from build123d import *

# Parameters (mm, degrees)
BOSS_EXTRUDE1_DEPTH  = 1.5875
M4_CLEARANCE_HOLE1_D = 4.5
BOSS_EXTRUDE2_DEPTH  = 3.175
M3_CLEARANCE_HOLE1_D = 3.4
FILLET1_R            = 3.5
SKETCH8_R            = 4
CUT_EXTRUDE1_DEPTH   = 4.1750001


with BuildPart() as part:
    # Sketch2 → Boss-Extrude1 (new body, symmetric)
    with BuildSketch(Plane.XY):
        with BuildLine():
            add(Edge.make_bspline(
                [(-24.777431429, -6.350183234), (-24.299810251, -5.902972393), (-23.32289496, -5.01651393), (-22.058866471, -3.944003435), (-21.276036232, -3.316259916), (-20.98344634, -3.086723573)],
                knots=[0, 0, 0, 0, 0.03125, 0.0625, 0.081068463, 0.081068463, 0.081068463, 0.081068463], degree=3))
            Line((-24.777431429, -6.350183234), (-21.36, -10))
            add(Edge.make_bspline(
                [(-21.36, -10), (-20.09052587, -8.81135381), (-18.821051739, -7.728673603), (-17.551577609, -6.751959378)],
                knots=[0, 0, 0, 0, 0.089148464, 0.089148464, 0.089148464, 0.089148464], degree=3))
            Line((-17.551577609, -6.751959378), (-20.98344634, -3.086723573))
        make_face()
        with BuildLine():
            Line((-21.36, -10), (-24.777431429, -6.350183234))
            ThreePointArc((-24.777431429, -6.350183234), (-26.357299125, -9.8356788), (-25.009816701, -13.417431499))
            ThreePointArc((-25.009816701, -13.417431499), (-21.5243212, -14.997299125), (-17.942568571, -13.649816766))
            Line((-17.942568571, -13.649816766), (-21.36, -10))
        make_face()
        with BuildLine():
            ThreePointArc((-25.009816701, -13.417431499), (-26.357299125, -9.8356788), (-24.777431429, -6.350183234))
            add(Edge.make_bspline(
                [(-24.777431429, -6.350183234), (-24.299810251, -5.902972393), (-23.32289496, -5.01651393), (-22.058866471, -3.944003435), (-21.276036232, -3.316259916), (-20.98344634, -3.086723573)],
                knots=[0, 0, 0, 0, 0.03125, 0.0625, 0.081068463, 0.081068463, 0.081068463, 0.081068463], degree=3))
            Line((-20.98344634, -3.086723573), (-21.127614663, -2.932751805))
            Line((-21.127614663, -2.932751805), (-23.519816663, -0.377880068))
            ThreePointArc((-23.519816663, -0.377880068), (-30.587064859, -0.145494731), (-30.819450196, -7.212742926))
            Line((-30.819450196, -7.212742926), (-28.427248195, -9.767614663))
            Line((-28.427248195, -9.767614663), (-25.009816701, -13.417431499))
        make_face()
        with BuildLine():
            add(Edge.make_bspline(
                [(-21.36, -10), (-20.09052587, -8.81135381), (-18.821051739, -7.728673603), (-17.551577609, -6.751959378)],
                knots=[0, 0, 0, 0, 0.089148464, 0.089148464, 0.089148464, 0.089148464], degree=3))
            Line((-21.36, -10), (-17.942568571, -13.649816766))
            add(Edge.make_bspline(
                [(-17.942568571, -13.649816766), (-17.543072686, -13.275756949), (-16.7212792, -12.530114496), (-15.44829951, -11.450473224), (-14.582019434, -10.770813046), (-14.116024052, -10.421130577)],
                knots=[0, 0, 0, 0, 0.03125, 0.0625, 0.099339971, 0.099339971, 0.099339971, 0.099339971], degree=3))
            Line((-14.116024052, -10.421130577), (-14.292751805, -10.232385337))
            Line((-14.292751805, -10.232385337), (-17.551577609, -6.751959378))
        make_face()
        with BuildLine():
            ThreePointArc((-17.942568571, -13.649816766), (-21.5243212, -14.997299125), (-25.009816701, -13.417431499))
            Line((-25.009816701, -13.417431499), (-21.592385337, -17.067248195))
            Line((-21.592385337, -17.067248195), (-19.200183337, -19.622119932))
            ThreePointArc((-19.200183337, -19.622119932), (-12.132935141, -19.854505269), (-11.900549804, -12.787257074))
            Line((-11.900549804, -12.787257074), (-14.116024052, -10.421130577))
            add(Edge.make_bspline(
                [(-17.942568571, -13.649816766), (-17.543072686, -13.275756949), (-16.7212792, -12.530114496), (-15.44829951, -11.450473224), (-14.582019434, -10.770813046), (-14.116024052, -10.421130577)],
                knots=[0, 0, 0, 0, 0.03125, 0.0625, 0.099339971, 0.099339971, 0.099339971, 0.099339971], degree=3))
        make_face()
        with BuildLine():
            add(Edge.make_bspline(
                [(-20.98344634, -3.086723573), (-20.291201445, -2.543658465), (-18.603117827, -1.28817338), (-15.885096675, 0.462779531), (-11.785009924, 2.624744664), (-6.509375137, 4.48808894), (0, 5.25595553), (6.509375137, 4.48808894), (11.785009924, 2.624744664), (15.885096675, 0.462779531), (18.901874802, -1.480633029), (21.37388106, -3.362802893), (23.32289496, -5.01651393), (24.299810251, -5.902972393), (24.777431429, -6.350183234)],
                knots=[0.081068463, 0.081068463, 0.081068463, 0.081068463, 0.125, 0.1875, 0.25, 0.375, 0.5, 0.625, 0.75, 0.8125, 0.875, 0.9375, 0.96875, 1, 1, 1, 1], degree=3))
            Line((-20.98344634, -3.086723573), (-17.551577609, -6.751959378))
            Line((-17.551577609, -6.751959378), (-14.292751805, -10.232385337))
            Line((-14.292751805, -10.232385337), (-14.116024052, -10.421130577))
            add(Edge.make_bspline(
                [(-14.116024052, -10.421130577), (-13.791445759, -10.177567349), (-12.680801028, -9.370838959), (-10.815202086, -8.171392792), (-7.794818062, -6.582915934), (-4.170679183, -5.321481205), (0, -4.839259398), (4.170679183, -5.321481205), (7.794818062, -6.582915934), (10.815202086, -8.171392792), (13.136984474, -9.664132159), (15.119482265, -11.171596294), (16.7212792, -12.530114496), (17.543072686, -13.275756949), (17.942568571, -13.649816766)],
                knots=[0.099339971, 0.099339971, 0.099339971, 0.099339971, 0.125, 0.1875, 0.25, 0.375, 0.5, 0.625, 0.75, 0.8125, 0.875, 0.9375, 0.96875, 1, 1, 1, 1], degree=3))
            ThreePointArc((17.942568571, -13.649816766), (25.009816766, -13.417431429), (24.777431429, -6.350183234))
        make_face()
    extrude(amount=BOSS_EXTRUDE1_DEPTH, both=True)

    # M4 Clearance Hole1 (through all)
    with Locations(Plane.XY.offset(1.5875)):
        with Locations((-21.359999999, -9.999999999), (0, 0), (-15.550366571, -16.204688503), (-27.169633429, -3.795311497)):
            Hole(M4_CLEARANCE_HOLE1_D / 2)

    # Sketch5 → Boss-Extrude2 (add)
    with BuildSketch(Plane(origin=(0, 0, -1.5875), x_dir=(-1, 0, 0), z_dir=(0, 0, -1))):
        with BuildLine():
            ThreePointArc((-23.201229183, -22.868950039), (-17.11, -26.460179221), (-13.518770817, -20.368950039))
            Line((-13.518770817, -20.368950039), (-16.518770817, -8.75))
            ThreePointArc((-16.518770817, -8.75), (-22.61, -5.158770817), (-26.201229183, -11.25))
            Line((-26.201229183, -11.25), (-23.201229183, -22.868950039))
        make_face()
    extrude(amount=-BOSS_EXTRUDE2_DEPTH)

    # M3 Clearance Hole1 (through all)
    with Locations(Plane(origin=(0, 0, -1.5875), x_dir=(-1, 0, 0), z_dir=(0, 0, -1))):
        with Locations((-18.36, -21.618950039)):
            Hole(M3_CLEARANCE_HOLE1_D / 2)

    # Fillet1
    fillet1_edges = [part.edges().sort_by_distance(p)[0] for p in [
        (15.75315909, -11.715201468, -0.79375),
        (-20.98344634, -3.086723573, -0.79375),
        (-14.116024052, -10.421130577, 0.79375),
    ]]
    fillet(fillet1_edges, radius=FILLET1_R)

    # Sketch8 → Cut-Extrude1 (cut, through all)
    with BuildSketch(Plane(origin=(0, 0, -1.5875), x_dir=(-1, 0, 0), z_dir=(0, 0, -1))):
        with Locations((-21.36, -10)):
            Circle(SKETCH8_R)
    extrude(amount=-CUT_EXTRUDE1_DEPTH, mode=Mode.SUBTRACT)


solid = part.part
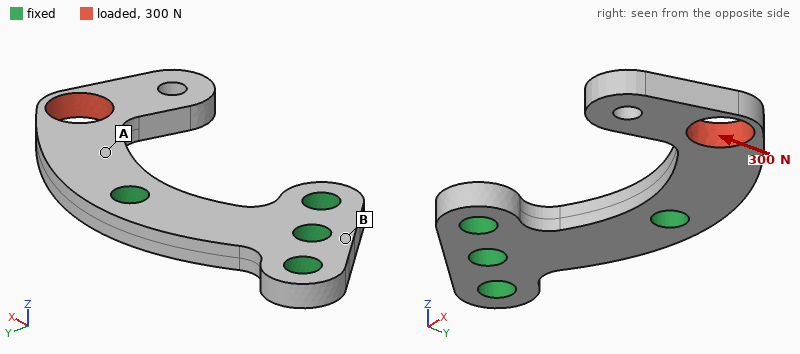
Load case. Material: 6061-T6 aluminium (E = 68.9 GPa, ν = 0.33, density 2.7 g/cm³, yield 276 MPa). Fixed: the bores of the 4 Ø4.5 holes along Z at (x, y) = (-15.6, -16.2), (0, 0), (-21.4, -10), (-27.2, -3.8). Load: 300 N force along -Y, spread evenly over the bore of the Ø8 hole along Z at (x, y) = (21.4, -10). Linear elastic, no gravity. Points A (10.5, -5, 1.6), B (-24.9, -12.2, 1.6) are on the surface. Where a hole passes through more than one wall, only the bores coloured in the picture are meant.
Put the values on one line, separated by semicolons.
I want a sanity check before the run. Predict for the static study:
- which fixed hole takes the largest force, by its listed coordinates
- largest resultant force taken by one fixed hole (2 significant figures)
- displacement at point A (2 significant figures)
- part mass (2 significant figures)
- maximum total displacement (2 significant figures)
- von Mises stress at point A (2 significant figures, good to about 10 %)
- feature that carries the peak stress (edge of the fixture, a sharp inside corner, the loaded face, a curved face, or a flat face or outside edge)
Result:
(0, 0); 390 N; 0.028 mm; 6.2 g; 0.17 mm; 28 MPa; edge of the fixture
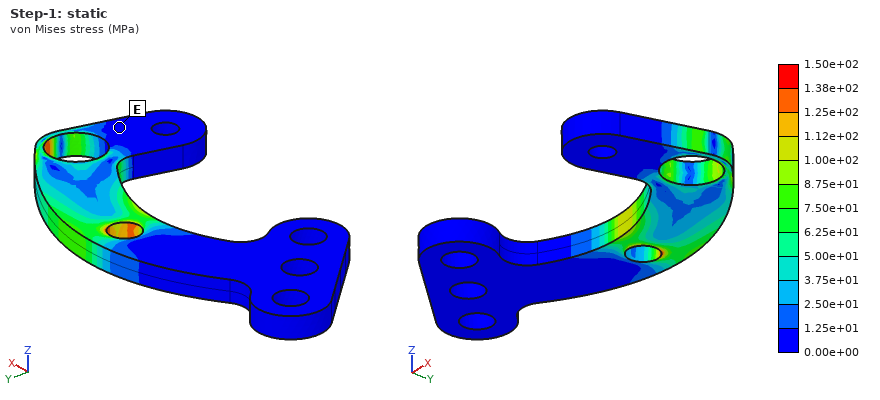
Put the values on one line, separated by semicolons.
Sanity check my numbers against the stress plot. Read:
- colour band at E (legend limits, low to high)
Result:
0.00e+00 to 1.25e+01 MPa
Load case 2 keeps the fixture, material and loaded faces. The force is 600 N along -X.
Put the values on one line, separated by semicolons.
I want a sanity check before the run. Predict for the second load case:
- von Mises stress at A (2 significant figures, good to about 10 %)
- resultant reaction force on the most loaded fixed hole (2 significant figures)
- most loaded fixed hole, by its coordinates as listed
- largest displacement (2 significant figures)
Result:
51 MPa; 580 N; (0, 0); 0.21 mm
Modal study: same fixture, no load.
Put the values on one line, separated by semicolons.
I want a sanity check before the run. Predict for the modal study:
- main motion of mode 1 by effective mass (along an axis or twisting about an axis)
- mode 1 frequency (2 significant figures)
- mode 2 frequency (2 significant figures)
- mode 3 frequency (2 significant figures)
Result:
along Z; 2300 Hz; 5300 Hz; 6700 Hz
